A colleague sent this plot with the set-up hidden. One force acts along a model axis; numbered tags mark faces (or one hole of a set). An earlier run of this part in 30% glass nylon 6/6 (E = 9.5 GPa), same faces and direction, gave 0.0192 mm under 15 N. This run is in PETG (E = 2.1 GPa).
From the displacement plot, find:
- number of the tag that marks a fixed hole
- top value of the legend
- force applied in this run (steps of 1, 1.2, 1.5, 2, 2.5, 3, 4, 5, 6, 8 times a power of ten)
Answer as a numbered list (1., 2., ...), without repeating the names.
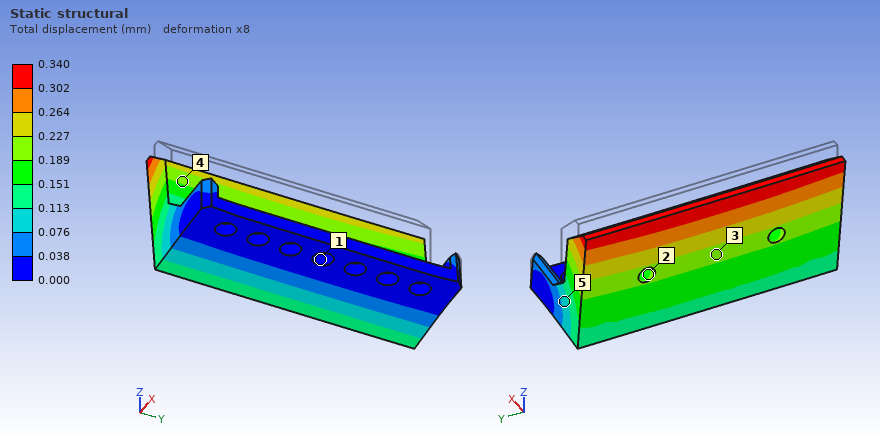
1. 1
2. 0.340 mm
3. 60 N
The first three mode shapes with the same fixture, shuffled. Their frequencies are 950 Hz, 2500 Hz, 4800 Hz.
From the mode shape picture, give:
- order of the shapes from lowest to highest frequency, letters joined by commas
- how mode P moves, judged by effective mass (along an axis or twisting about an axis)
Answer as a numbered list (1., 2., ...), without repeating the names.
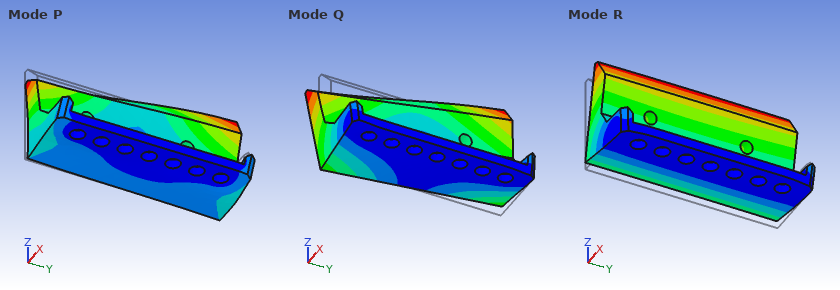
1. R, Q, P
2. along Y
